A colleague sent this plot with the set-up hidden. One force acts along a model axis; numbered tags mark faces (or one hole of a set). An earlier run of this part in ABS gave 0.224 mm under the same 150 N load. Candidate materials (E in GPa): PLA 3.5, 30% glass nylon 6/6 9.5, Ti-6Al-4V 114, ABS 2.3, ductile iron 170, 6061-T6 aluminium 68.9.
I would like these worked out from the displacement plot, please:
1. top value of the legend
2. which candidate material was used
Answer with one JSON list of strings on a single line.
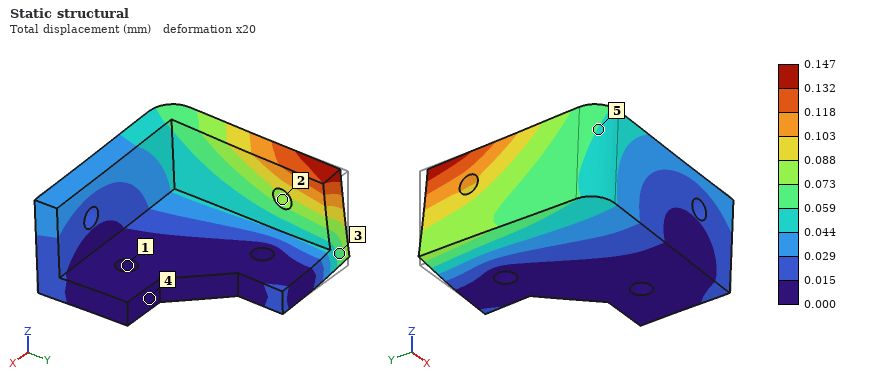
["0.147 mm", "PLA"]
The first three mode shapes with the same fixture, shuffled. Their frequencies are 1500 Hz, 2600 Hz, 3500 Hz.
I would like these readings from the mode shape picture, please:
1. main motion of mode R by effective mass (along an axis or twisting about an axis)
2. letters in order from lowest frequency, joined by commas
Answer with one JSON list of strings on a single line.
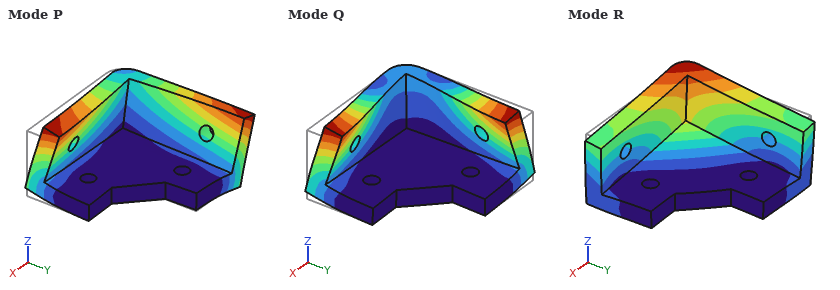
["along Z", "R, P, Q"]
